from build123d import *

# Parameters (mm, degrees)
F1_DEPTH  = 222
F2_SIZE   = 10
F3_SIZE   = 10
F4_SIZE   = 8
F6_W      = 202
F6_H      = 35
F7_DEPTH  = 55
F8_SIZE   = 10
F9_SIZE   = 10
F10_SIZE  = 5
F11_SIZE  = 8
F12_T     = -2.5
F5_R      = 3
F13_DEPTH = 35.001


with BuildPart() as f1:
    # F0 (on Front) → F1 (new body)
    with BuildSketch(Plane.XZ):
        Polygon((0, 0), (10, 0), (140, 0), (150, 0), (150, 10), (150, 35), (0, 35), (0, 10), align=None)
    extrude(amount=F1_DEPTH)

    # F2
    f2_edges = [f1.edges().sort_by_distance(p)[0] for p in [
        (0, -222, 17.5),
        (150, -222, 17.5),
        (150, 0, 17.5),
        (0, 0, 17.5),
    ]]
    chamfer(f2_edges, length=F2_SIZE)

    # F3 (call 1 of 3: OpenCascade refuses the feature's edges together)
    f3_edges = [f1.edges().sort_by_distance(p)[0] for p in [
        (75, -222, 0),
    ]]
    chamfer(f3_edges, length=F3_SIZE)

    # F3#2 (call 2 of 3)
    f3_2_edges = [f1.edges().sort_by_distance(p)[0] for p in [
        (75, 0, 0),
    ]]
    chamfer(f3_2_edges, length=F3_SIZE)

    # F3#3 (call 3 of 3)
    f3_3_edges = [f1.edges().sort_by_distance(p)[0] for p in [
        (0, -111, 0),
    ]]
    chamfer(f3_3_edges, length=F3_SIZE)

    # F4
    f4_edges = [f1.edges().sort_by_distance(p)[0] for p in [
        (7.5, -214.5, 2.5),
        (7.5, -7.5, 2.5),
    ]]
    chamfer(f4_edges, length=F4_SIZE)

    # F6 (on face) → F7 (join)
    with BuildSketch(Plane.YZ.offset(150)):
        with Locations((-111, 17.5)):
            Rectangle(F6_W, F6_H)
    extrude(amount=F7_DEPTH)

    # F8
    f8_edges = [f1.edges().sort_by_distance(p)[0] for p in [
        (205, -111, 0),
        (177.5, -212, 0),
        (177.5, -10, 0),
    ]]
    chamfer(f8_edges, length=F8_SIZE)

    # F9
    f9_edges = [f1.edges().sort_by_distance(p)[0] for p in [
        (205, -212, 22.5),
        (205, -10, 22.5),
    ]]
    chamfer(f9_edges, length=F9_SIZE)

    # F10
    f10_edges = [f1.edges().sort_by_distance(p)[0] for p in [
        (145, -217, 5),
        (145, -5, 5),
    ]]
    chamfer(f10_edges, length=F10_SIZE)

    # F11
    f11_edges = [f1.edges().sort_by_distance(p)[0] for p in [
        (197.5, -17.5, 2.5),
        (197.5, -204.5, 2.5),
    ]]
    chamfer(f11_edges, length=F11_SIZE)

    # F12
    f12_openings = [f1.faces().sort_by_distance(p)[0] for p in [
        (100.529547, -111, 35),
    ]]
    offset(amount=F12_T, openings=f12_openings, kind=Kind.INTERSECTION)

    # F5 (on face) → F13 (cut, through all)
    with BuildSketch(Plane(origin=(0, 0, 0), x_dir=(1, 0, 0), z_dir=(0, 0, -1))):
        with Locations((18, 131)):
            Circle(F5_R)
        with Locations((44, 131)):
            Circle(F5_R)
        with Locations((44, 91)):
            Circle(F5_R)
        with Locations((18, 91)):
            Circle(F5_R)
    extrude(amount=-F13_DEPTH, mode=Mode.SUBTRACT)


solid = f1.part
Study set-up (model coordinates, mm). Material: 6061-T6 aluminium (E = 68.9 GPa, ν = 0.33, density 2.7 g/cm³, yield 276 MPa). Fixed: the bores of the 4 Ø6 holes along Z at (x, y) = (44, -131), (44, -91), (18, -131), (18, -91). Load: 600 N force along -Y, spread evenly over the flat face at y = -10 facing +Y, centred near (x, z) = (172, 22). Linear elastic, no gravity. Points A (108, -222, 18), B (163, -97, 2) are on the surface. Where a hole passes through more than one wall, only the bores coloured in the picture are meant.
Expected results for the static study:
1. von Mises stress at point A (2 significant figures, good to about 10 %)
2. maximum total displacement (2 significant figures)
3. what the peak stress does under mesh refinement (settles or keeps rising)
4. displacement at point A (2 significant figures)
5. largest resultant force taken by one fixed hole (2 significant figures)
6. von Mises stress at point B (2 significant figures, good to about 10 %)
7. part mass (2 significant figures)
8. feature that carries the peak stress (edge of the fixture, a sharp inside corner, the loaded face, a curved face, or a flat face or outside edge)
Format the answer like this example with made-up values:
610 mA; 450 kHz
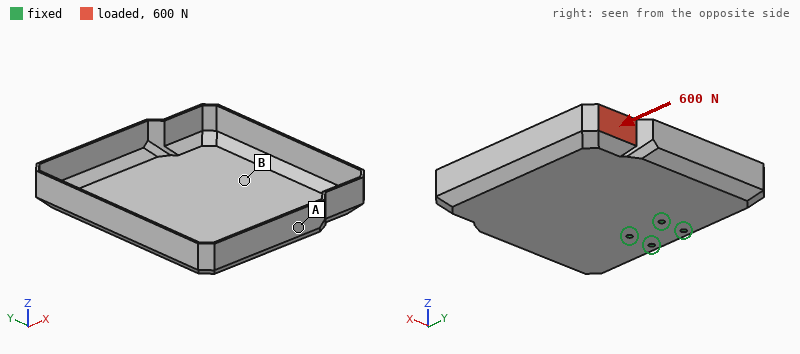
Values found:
19 MPa; 3.6 mm; keeps rising; 1.7 mm; 1.2 kN; 27 MPa; 440 g; edge of the fixture
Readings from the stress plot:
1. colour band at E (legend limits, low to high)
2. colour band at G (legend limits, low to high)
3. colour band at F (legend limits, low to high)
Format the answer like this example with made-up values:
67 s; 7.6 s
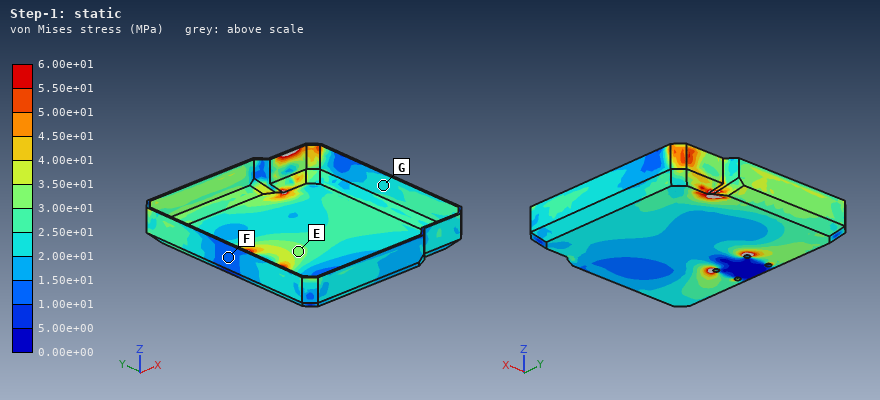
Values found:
3.00e+01 to 3.50e+01 MPa; 2.00e+01 to 2.50e+01 MPa; 1.00e+01 to 1.50e+01 MPa
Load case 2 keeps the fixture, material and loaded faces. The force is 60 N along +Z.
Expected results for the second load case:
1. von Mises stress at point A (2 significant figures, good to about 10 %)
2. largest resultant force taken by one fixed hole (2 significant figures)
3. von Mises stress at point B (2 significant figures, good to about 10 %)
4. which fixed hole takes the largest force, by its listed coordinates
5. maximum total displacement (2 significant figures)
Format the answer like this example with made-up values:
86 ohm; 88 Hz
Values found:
12 MPa; 180 N; 8.8 MPa; (44, -91); 3.0 mm
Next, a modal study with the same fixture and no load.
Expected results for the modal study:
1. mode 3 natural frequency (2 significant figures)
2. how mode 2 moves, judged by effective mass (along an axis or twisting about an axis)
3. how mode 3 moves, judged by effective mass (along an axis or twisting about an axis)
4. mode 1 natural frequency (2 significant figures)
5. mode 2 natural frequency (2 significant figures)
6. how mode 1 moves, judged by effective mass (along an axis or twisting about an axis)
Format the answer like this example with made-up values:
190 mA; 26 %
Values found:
530 Hz; twisting about X; twisting about X; 77 Hz; 110 Hz; along Z
